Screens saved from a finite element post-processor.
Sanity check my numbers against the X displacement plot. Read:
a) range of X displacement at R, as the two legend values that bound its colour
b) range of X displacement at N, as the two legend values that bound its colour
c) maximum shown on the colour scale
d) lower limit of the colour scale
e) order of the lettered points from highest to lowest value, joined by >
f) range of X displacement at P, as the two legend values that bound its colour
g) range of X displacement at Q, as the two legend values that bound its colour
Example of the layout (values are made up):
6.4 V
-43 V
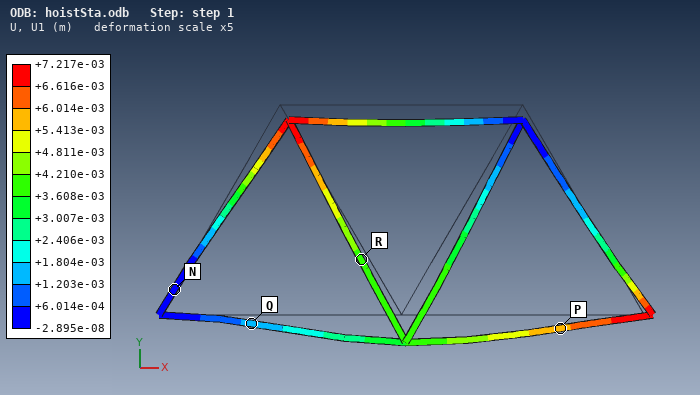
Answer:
+3.608e-03 to +4.210e-03 m
-2.895e-08 to +6.014e-04 m
+7.217e-03 m
-2.895e-08 m
P > R > Q > N
+5.413e-03 to +6.014e-03 m
+1.203e-03 to +1.804e-03 m
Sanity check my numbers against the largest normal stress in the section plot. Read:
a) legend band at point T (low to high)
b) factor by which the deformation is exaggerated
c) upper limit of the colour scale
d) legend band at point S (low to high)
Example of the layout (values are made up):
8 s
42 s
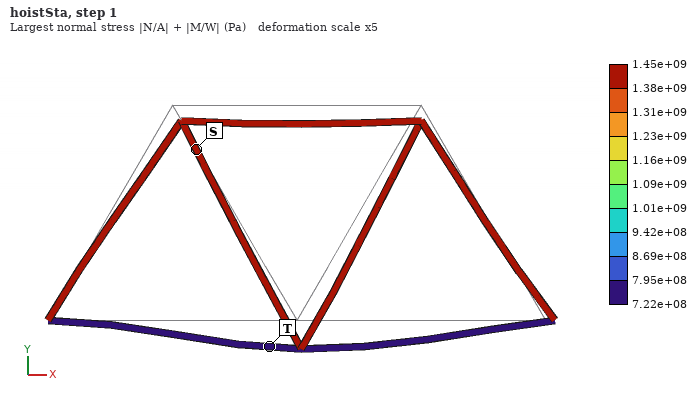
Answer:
7.22e+08 to 7.95e+08 Pa
5
1.45e+09 Pa
1.38e+09 to 1.45e+09 Pa
